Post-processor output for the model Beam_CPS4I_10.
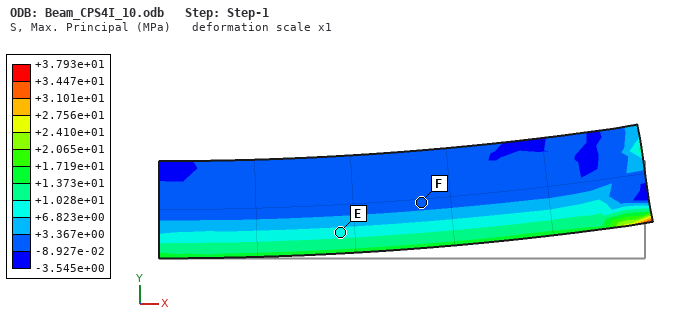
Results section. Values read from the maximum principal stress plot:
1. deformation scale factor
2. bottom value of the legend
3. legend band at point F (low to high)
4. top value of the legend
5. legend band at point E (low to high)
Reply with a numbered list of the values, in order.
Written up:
1. 1
2. -3.545e+00 MPa
3. -8.927e-02 to +3.367e+00 MPa
4. +3.793e+01 MPa
5. +6.823e+00 to +1.028e+01 MPa
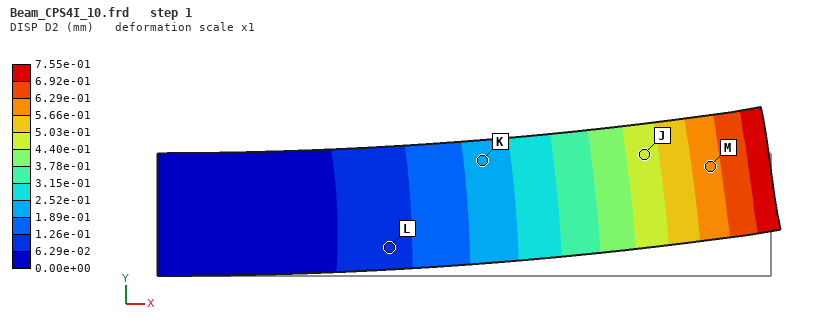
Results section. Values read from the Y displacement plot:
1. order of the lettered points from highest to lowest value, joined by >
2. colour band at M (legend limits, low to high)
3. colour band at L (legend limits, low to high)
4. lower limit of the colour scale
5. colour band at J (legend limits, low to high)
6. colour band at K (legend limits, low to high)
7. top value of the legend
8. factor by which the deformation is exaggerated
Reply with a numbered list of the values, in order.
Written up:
1. M > J > K > L
2. 5.66e-01 to 6.29e-01 mm
3. 6.29e-02 to 1.26e-01 mm
4. 0.00e+00 mm
5. 4.40e-01 to 5.03e-01 mm
6. 1.89e-01 to 2.52e-01 mm
7. 7.55e-01 mm
8. 1
